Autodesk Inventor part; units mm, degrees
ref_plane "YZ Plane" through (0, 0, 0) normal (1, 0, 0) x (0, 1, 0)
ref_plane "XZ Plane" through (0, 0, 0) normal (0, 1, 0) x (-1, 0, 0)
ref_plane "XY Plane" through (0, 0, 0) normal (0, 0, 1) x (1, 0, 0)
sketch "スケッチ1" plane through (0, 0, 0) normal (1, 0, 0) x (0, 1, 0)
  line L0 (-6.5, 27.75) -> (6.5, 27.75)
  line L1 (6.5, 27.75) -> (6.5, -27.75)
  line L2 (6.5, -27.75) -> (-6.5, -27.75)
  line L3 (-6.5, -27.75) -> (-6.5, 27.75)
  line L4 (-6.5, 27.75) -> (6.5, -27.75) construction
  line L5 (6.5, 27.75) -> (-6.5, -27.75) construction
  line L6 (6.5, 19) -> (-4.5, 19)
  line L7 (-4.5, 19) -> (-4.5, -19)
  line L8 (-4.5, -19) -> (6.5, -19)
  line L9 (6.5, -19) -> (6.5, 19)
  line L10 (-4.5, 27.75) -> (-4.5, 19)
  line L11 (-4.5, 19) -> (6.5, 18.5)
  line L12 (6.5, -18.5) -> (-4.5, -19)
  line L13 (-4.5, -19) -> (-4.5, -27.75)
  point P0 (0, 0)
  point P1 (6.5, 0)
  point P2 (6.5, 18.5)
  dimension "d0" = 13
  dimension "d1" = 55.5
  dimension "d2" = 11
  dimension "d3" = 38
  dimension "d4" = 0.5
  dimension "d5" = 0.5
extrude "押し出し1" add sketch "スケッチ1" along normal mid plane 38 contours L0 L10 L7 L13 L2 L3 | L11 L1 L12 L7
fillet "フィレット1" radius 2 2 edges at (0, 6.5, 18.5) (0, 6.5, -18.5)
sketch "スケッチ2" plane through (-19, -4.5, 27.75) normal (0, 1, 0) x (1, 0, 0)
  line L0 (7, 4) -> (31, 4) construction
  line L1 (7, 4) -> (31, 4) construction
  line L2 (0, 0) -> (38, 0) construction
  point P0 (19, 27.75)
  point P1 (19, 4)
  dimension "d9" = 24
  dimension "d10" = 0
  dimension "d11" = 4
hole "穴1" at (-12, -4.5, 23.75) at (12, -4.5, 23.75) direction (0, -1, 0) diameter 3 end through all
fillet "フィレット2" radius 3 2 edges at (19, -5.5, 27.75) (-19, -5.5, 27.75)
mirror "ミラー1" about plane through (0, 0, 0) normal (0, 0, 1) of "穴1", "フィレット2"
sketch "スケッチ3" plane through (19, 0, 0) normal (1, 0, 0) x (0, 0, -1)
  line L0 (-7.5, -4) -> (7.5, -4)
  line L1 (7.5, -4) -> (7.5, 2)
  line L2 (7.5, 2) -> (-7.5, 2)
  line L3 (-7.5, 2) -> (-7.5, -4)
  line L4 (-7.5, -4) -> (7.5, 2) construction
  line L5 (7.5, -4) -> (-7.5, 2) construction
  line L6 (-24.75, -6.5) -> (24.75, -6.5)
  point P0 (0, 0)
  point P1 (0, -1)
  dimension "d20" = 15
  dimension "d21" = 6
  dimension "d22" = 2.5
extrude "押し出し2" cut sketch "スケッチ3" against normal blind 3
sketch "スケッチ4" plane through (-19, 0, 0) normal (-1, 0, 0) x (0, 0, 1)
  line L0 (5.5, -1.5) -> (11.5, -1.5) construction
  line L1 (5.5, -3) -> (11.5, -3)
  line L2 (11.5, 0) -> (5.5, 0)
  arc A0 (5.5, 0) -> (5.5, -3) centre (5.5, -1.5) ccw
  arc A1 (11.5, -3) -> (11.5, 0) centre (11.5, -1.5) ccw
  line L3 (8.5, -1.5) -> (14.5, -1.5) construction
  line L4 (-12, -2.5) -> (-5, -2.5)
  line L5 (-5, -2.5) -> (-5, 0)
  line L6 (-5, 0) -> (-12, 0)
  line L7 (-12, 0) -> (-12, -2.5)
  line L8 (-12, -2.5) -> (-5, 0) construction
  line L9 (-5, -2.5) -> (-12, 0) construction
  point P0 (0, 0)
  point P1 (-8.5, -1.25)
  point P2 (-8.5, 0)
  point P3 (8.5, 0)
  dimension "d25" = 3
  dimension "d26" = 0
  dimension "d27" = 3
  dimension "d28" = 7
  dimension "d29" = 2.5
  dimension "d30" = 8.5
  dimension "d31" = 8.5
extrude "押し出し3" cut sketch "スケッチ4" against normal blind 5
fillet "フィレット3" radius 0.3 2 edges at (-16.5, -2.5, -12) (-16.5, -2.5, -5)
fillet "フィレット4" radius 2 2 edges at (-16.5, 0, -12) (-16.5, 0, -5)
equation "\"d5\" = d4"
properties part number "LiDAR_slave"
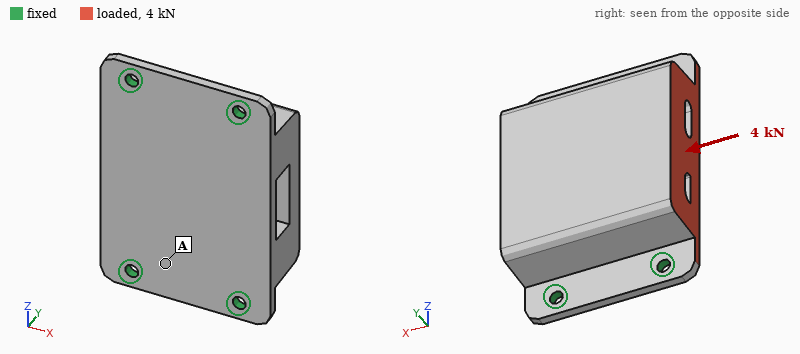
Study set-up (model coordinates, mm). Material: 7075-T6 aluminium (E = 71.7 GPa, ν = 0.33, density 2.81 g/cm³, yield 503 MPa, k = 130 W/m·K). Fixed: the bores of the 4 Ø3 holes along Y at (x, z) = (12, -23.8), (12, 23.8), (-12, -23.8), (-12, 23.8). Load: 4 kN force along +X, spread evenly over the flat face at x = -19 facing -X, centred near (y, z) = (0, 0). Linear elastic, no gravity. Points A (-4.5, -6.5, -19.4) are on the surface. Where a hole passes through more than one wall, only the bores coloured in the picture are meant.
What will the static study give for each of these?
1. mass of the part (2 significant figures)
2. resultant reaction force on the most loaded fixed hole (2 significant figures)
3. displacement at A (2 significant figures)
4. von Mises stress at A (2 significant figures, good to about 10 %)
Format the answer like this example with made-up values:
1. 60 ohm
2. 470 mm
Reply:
1. 54 g
2. 1.2 kN
3. 7.3 µm
4. 31 MPa
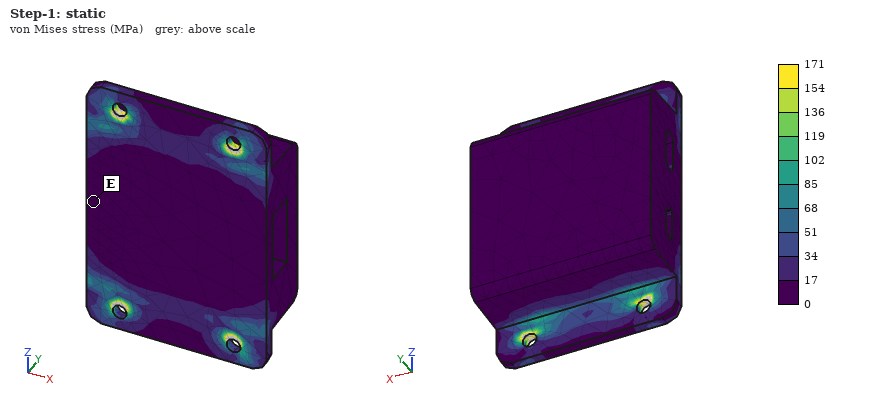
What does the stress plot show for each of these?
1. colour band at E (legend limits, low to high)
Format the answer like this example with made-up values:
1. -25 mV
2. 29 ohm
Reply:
1. 0 to 17 MPa
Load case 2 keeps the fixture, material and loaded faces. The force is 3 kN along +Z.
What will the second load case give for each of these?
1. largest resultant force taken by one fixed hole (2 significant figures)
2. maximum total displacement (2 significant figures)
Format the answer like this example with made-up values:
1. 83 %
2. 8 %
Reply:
1. 1.2 kN
2. 15 µm
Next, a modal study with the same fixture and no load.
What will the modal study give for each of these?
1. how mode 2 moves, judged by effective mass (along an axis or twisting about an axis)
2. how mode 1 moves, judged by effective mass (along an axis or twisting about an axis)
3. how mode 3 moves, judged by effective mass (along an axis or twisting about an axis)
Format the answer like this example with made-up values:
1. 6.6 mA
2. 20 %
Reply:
1. along Y
2. along X
3. along Z
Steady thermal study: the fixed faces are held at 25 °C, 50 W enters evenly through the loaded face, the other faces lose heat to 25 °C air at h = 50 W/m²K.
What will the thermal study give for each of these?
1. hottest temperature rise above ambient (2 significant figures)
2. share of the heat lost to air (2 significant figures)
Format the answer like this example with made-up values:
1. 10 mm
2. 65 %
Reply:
1. 32 K
2. 11 %
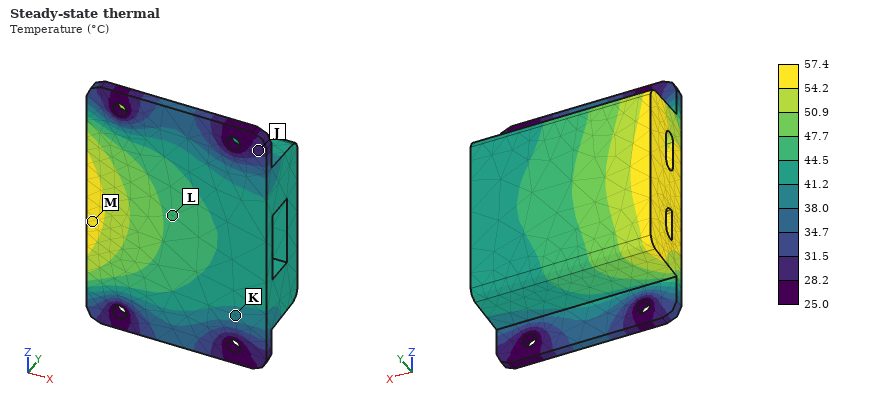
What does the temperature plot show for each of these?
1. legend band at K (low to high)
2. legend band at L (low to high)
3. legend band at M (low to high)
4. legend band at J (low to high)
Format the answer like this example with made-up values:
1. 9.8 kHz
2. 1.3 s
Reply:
1. 38.0 to 41.2 °C
2. 44.5 to 47.7 °C
3. 54.2 to 57.4 °C
4. 28.2 to 31.5 °C
